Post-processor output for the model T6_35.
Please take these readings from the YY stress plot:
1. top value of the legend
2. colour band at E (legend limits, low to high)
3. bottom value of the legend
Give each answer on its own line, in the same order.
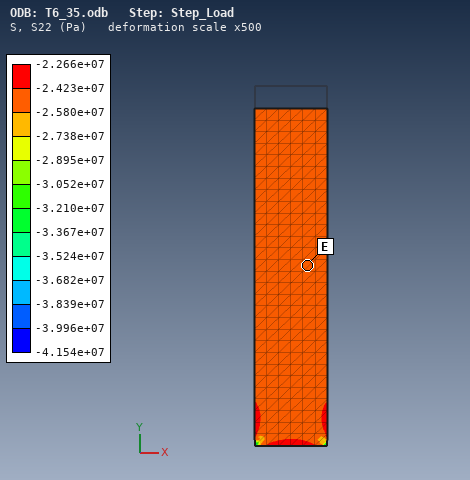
-2.266e+07 Pa
-2.580e+07 to -2.423e+07 Pa
-4.154e+07 Pa
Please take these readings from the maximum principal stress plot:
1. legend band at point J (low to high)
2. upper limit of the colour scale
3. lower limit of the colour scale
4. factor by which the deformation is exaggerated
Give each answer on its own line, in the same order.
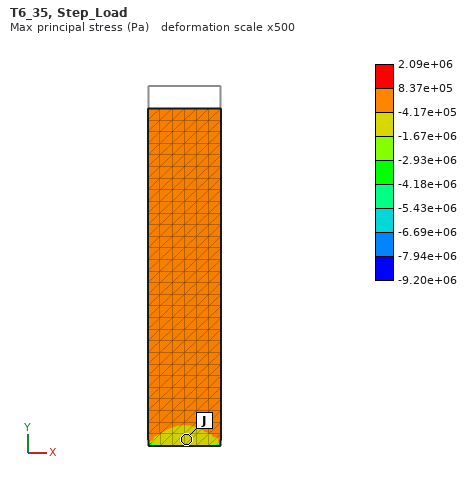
-1.67e+06 to -4.17e+05 Pa
2.09e+06 Pa
-9.20e+06 Pa
500
